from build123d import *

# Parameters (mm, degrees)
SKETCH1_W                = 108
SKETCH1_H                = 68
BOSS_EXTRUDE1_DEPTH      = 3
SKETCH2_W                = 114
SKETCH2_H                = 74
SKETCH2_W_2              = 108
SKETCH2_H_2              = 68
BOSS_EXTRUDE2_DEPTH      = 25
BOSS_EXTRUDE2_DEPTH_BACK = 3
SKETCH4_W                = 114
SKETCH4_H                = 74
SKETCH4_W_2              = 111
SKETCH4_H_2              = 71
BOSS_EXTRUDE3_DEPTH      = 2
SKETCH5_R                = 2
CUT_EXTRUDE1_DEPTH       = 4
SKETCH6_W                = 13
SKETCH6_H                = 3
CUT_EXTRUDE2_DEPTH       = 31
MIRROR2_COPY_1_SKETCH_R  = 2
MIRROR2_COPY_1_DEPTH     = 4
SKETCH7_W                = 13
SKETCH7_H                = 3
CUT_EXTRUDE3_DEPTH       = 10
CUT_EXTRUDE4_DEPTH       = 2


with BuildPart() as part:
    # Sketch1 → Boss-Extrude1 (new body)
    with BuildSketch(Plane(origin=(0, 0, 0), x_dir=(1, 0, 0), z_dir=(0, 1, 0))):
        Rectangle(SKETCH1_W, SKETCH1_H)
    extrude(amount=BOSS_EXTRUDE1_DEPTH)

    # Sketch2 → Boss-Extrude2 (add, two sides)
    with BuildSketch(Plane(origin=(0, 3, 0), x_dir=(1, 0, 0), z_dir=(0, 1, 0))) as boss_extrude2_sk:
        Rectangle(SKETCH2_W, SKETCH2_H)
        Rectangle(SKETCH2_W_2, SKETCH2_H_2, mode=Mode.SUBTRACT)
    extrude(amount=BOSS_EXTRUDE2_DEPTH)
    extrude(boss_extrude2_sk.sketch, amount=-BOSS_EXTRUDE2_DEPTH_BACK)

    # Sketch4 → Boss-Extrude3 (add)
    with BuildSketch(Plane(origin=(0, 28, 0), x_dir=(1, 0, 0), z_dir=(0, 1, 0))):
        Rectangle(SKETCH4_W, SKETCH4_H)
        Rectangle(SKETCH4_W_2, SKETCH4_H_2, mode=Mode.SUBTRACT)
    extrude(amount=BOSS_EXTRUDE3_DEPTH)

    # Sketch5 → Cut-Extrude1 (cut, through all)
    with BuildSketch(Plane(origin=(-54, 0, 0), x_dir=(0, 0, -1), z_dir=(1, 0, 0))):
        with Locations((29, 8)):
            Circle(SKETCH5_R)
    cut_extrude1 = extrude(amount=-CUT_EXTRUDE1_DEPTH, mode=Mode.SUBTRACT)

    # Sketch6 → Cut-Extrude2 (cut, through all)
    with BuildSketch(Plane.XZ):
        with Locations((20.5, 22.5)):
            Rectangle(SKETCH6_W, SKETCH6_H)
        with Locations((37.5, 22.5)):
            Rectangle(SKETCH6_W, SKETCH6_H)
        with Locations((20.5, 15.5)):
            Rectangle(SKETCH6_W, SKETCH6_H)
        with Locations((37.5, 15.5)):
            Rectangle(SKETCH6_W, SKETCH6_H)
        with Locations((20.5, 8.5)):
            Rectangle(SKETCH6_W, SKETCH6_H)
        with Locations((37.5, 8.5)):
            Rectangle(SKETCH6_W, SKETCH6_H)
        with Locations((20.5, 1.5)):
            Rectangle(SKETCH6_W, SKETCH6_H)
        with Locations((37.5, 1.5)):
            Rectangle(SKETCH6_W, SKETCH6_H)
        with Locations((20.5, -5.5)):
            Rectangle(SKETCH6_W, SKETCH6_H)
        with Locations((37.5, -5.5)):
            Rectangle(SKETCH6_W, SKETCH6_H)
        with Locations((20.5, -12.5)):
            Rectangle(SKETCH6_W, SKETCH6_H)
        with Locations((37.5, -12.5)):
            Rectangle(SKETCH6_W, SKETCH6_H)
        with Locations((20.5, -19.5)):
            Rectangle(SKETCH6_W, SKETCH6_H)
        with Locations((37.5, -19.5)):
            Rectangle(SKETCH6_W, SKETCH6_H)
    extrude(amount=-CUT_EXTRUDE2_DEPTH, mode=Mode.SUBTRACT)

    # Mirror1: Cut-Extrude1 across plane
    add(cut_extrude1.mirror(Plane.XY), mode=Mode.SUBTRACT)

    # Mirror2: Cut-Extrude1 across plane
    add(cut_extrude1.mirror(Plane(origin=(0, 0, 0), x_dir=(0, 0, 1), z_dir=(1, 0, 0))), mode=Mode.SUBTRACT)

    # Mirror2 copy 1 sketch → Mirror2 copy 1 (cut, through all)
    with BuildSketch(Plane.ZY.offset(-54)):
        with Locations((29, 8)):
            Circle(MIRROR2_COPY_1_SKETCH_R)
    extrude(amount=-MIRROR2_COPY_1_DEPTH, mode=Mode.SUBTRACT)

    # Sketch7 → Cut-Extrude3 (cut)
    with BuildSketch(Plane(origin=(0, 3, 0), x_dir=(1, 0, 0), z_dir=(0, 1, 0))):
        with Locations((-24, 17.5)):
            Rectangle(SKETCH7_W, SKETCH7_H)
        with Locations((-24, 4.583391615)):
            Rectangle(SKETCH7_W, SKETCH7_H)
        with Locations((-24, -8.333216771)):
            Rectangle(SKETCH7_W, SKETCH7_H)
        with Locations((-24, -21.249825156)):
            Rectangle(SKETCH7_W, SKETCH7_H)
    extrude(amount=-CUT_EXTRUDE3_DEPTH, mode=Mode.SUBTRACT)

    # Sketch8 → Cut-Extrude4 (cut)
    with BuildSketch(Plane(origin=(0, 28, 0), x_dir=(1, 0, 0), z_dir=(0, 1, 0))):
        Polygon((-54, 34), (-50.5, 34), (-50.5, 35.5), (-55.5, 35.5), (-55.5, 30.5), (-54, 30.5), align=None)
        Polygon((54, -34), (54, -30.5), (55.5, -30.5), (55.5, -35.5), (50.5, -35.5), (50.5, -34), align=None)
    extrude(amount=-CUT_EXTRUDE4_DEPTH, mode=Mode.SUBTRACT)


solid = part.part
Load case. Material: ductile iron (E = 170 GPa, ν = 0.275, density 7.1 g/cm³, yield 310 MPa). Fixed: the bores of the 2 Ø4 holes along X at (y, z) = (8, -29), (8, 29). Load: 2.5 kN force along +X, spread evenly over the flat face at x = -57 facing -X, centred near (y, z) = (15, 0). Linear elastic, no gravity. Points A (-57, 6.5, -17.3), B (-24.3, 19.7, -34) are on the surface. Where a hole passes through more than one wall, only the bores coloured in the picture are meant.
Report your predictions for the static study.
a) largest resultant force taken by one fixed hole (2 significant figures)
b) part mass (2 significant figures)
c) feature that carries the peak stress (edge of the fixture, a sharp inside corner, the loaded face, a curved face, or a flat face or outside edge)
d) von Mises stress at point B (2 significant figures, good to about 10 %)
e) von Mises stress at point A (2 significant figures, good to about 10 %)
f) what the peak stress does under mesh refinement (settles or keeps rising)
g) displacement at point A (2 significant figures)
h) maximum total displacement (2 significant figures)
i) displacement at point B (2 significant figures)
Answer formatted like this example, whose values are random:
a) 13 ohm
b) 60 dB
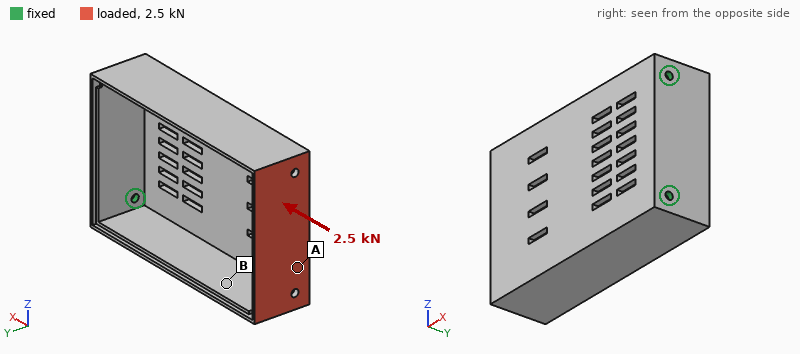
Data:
a) 1.3 kN
b) 370 g
c) edge of the fixture
d) 17 MPa
e) 84 MPa
f) keeps rising
g) 0.35 mm
h) 0.45 mm
i) 0.24 mm
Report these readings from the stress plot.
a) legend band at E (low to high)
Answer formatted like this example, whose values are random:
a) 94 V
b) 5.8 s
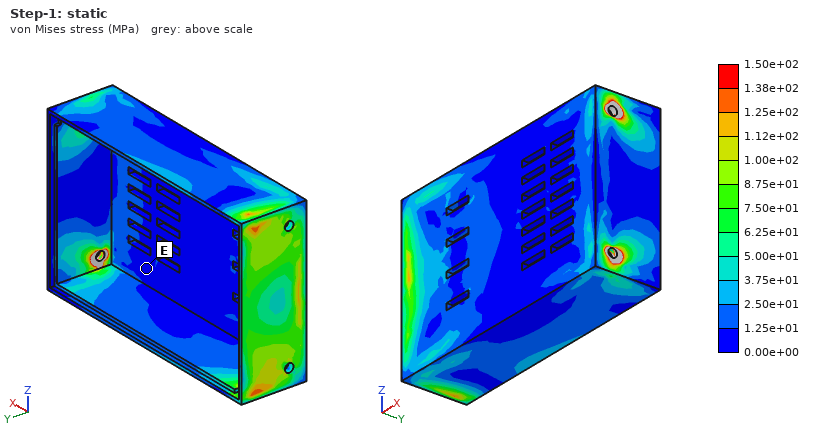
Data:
a) 0.00e+00 to 1.25e+01 MPa
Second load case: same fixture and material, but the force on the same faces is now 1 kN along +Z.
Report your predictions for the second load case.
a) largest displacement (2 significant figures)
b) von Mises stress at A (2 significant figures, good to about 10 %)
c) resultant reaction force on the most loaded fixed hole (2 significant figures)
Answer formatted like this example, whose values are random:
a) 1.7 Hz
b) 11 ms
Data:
a) 0.65 mm
b) 41 MPa
c) 1.9 kN
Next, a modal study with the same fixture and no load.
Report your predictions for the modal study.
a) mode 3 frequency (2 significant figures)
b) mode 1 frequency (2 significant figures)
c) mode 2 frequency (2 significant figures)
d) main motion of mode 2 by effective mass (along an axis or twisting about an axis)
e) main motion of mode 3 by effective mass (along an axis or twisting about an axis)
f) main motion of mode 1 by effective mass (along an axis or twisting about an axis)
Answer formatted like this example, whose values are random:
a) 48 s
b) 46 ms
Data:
a) 1700 Hz
b) 320 Hz
c) 540 Hz
d) along Z
e) along Z
f) along Y
